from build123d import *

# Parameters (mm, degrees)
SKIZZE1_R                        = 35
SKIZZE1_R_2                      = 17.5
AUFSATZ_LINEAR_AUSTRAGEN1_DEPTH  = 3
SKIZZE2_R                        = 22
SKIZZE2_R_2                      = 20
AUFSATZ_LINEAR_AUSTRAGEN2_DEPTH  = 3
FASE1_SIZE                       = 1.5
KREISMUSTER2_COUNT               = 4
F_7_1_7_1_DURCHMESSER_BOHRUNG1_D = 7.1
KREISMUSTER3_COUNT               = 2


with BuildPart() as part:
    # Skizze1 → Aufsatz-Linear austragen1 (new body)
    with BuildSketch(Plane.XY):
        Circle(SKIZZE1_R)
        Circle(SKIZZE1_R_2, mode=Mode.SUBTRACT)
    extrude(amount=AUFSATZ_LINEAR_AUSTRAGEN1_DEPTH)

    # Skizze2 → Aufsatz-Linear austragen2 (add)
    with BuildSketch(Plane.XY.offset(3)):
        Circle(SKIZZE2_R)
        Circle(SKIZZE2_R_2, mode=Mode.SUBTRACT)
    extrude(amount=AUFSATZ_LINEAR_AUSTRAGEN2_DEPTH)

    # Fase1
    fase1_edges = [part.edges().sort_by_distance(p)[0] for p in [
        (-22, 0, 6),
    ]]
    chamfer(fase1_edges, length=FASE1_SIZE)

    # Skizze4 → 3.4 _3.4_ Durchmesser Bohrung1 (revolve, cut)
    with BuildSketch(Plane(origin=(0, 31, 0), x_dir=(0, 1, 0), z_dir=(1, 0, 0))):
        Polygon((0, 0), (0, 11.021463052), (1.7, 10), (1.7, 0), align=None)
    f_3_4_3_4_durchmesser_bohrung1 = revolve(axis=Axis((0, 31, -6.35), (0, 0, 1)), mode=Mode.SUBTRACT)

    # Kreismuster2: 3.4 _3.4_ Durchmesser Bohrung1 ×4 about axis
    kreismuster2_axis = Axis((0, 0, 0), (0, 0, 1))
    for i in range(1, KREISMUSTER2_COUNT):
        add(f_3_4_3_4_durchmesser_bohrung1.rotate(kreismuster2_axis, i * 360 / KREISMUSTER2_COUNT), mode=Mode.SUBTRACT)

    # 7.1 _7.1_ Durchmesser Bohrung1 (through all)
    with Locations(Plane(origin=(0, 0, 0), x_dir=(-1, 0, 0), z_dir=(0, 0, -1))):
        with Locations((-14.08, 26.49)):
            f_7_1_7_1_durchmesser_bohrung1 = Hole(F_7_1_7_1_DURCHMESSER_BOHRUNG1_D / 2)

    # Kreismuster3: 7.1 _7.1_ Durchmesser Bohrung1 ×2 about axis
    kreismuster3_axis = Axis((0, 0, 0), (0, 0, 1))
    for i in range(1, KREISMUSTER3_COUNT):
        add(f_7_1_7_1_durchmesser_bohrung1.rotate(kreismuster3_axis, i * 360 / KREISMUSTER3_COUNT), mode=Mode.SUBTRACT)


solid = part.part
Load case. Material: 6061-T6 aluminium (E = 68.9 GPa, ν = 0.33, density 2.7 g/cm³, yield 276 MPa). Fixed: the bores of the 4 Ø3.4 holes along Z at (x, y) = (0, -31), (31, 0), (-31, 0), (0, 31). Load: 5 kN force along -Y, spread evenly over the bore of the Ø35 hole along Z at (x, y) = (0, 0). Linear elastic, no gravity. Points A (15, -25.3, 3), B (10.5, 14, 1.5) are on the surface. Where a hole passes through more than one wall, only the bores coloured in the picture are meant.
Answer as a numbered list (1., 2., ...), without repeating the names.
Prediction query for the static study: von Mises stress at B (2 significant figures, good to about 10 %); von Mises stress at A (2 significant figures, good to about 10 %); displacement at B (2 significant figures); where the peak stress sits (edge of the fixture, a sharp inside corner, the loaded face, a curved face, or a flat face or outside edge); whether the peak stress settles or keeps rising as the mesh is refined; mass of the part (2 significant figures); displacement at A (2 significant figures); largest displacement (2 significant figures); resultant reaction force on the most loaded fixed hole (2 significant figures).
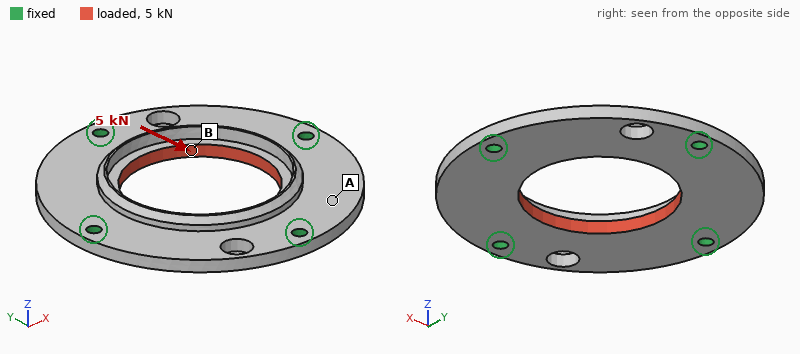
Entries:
1. 25 MPa
2. 11 MPa
3. 12 µm
4. edge of the fixture
5. keeps rising
6. 24 g
7. 8.1 µm
8. 13 µm
9. 1.3 kN
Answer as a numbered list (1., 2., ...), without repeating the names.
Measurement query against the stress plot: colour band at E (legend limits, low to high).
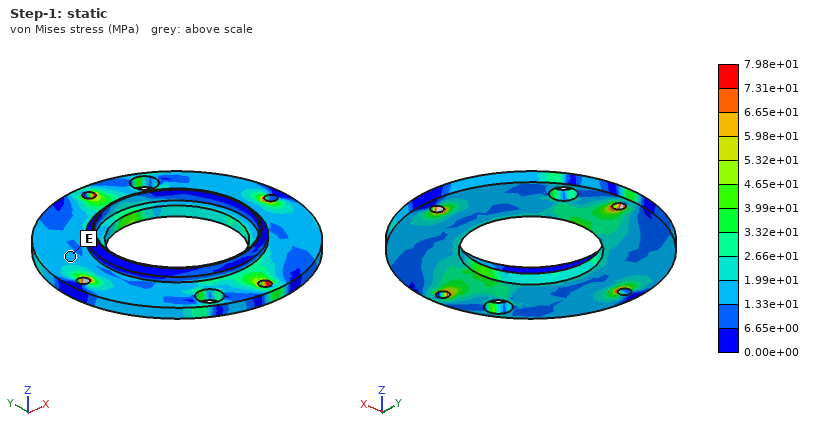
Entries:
1. 1.33e+01 to 1.99e+01 MPa
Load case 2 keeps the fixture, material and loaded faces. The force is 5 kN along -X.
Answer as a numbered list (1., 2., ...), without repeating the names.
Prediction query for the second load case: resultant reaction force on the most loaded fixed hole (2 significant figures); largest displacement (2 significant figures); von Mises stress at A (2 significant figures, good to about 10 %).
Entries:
1. 1.3 kN
2. 14 µm
3. 17 MPa
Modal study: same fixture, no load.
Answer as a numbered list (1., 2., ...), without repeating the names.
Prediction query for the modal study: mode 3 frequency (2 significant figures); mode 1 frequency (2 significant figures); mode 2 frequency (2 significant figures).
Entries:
1. 7600 Hz
2. 6800 Hz
3. 7400 Hz
